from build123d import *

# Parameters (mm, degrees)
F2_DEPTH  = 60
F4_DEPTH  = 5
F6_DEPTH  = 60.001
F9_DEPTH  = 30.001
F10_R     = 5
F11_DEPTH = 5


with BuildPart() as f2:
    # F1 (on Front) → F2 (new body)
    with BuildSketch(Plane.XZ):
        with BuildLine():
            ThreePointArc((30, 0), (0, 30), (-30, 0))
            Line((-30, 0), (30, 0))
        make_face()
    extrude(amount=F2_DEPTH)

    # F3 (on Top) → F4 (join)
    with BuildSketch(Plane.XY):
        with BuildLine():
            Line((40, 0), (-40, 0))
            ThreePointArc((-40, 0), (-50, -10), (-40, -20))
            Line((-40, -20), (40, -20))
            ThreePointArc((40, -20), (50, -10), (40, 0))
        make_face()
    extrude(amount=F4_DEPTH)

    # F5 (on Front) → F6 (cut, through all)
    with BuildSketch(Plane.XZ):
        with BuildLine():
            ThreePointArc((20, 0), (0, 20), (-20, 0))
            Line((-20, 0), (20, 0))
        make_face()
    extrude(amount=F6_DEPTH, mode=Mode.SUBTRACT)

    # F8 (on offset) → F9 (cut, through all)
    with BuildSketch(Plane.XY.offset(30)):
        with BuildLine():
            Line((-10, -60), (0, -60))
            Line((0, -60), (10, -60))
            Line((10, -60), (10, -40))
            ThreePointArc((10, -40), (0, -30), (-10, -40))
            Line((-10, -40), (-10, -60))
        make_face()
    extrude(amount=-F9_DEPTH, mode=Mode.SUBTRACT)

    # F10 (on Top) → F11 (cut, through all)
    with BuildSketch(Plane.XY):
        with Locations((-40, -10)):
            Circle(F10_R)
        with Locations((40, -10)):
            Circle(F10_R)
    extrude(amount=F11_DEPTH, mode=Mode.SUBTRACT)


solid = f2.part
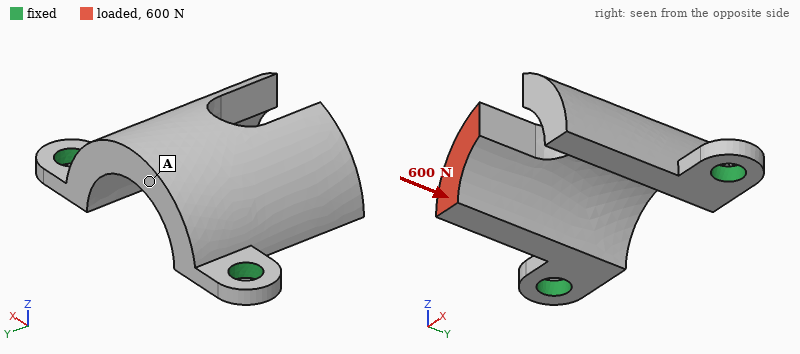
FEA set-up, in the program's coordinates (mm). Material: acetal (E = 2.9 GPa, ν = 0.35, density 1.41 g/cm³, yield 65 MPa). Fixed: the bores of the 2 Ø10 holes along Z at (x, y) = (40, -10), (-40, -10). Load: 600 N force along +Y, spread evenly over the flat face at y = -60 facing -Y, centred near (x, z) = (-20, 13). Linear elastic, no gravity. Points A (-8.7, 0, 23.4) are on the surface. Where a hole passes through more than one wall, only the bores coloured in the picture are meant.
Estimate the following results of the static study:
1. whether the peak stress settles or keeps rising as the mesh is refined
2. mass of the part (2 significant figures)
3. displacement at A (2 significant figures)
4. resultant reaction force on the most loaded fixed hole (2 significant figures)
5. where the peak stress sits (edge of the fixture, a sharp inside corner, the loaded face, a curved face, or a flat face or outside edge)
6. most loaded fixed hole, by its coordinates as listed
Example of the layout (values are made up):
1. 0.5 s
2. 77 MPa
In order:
1. keeps rising
2. 62 g
3. 0.61 mm
4. 480 N
5. edge of the fixture
6. (-40, -10)
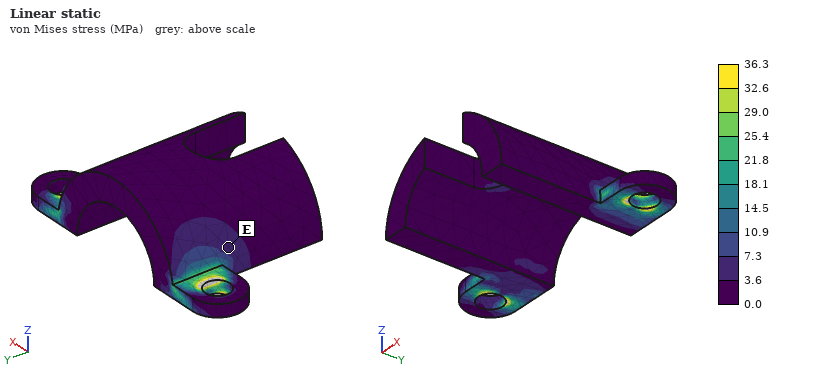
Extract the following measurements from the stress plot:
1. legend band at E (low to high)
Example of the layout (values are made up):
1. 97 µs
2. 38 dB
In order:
1. 3.6 to 7.3 MPa
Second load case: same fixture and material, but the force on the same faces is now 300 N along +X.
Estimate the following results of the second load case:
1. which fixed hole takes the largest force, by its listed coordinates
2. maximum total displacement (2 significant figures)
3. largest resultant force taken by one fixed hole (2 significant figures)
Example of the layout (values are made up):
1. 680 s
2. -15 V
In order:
1. (-40, -10)
2. 1.2 mm
3. 260 N
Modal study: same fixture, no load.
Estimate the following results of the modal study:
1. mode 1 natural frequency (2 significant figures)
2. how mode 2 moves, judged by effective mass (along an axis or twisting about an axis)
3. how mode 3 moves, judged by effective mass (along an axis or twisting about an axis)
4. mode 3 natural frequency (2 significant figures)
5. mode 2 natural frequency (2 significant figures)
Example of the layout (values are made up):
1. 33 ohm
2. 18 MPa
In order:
1. 380 Hz
2. along X
3. along Y
4. 1300 Hz
5. 850 Hz
